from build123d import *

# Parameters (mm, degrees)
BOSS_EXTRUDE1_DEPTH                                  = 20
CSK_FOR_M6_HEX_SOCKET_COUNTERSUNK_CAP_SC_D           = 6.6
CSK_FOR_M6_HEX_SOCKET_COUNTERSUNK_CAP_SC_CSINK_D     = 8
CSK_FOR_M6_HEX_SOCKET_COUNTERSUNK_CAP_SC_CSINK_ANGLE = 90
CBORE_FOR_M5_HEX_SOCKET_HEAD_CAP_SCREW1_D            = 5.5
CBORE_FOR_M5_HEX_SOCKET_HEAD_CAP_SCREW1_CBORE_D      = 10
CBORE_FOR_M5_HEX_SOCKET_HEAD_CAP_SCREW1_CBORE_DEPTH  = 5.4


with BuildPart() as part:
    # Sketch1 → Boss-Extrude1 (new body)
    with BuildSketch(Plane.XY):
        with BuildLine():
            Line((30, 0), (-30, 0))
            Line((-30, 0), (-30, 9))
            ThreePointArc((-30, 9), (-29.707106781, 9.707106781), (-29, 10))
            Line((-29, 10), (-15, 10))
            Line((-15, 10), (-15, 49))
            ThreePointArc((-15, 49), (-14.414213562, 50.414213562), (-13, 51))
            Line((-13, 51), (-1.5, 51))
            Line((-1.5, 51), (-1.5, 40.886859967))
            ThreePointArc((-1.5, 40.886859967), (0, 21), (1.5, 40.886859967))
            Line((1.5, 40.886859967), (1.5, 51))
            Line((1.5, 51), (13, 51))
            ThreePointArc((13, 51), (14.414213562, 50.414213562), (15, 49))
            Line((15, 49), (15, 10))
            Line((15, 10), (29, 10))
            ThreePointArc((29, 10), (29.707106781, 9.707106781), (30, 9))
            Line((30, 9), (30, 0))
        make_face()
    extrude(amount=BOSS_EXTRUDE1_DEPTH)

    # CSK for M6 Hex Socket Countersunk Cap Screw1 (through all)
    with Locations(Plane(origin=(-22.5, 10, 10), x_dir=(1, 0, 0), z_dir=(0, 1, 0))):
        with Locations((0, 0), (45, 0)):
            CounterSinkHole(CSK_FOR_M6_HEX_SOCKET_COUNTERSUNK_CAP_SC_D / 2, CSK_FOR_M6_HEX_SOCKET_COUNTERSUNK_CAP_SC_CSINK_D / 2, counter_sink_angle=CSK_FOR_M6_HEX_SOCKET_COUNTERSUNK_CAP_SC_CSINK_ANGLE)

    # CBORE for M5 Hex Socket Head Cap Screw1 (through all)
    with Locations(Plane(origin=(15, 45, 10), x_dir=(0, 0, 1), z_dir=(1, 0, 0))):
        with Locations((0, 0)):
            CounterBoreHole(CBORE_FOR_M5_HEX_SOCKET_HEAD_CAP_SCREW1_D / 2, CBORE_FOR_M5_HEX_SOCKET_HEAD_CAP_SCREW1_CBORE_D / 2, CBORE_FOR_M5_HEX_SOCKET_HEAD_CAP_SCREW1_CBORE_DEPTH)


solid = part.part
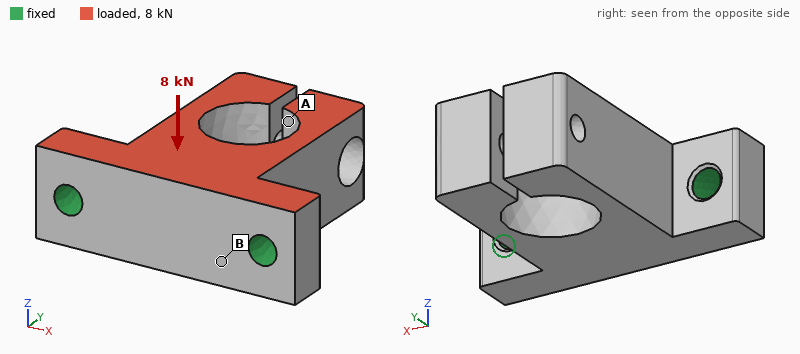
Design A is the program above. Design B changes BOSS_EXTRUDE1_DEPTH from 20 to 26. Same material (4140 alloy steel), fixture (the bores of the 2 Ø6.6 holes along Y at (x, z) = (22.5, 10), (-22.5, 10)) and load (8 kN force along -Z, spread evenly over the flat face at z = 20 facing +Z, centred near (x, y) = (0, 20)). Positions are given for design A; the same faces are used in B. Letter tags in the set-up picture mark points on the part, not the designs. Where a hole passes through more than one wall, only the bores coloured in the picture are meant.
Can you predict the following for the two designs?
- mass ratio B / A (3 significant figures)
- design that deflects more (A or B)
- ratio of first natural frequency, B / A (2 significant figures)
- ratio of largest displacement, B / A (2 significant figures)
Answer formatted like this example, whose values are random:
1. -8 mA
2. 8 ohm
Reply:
1. 1.32
2. A
3. 0.99
4. 0.73
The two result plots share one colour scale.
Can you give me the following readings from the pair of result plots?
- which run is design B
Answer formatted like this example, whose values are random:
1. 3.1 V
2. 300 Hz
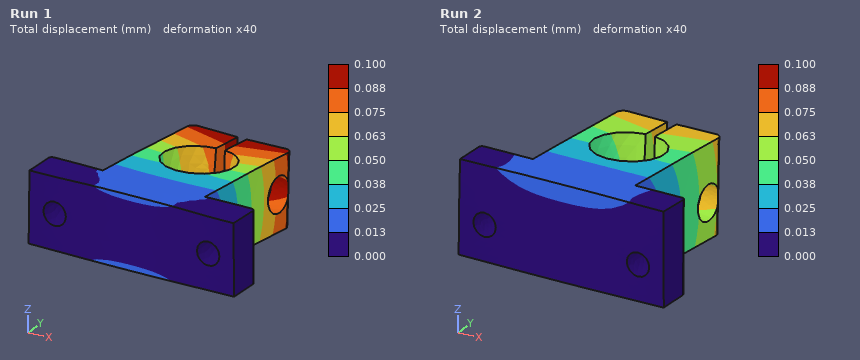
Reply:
1. Run 2
